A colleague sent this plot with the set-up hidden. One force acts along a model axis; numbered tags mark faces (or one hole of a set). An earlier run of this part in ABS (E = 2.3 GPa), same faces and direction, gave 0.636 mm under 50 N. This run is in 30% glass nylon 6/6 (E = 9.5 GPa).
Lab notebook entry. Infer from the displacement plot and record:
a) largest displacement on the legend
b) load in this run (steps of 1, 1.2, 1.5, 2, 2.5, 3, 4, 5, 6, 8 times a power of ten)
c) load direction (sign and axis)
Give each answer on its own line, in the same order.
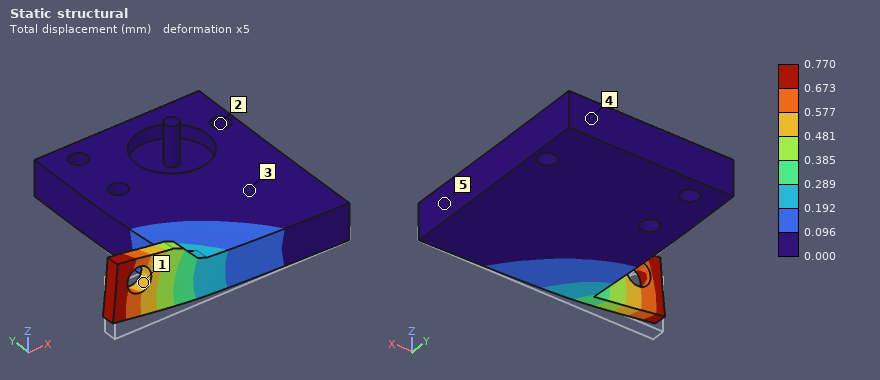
0.770 mm
250 N
+Z
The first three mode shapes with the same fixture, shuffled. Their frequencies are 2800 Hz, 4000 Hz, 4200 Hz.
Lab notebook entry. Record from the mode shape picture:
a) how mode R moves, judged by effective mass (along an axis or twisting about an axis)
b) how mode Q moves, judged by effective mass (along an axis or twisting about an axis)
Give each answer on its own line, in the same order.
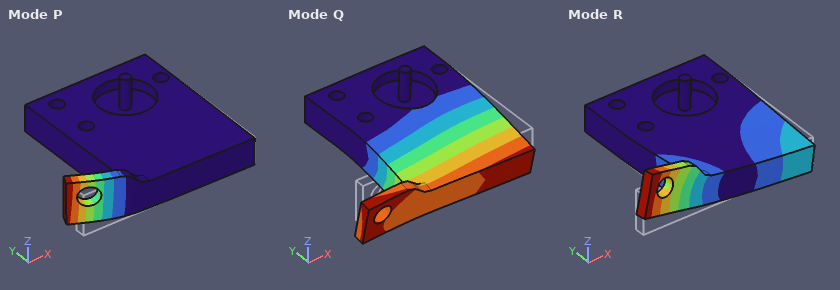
twisting about Y
along Z
